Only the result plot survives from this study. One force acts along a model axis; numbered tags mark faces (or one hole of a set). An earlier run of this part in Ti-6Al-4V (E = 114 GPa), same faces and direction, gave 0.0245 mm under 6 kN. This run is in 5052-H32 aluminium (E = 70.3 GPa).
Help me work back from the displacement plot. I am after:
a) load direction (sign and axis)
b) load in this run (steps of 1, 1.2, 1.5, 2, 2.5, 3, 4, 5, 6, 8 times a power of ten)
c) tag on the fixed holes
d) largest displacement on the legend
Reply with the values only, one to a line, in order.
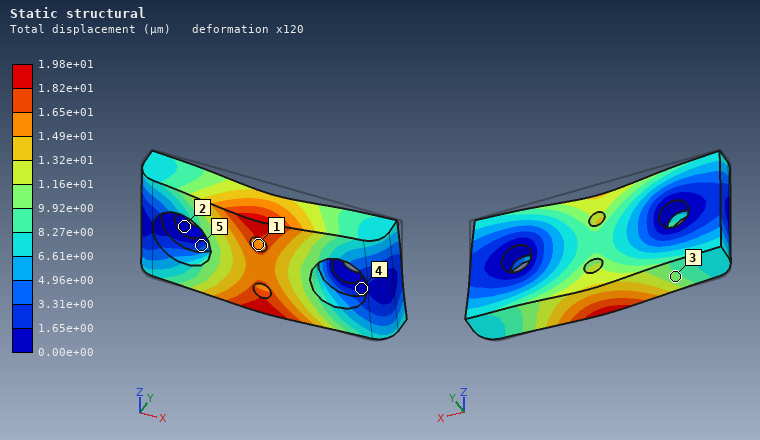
-Z
3 kN
2
1.98e+01 µm
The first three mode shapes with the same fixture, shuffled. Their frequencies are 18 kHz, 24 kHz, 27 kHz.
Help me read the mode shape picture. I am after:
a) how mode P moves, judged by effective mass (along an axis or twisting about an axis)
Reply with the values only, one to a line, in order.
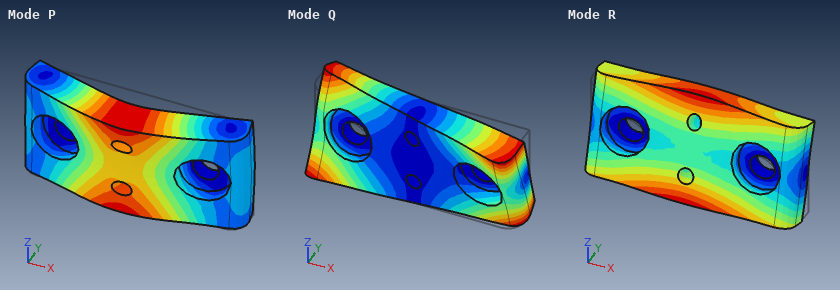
along Y
